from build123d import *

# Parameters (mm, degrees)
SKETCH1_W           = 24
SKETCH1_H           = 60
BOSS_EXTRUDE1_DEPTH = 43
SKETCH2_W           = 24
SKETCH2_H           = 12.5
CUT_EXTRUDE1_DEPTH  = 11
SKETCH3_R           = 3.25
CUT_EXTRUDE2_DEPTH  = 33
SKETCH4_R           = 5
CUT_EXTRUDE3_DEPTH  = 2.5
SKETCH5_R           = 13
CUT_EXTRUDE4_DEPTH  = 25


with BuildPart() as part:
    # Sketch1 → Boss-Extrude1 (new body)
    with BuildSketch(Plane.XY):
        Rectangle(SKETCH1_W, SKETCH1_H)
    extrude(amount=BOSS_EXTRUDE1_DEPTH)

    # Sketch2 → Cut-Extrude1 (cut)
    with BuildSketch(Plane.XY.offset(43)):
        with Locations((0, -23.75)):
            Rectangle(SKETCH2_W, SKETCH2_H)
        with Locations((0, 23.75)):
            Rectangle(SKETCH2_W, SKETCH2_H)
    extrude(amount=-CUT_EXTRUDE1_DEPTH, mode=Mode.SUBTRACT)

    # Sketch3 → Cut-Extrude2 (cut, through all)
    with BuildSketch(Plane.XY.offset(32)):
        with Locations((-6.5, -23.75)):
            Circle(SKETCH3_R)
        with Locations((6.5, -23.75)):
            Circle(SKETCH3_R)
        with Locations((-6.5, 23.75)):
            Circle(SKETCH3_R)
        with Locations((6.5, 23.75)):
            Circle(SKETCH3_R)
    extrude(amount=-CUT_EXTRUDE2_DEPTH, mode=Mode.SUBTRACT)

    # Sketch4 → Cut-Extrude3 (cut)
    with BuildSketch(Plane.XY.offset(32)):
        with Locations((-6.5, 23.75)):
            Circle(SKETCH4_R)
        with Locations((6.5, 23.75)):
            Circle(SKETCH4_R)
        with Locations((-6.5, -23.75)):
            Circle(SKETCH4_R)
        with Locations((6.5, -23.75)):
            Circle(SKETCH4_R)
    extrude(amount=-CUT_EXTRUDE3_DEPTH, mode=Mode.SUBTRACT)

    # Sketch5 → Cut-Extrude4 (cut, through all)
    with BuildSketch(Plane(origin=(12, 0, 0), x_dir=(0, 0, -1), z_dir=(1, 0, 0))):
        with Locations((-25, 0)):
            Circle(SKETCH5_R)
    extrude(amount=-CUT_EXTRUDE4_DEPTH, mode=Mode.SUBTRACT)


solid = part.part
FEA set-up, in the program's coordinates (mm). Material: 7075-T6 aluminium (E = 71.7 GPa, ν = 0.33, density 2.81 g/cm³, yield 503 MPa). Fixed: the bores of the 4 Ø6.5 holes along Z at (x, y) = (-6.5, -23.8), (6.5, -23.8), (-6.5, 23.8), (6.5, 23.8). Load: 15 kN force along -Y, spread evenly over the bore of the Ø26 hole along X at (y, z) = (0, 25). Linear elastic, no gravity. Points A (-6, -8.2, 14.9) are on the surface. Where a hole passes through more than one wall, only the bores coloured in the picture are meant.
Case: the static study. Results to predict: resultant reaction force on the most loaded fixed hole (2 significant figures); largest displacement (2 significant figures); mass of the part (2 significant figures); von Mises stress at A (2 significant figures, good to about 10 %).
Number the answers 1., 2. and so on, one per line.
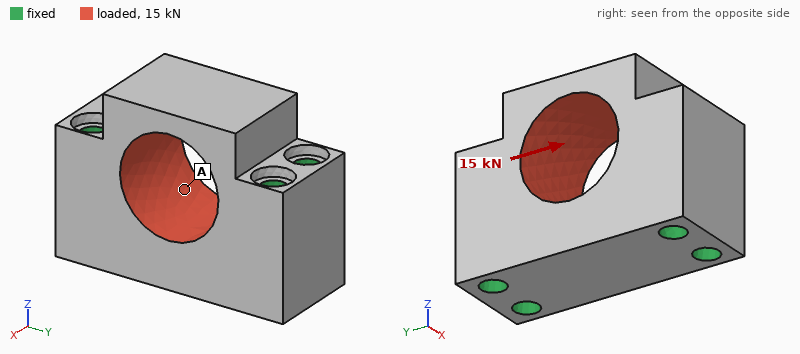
1. 3.9 kN
2. 16 µm
3. 110 g
4. 11 MPa
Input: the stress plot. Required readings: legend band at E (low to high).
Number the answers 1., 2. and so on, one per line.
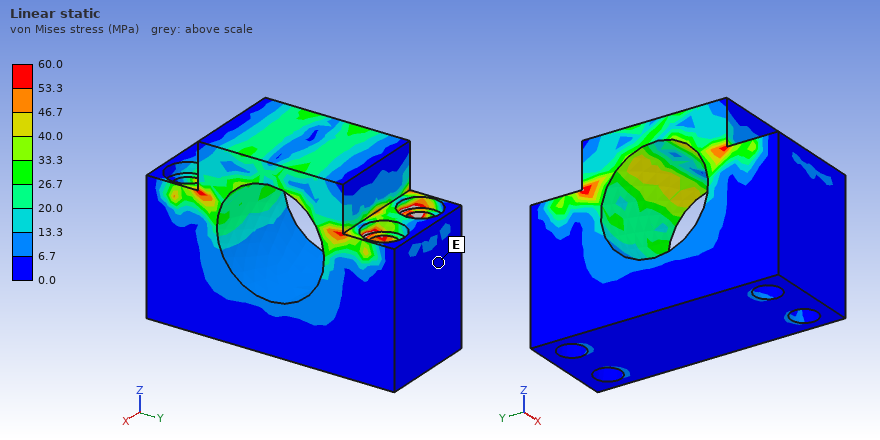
1. 0.0 to 6.7 MPa
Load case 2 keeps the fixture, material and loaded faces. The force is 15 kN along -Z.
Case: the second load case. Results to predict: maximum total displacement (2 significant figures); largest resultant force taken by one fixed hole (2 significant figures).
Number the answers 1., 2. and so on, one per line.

1. 14 µm
2. 3.8 kN
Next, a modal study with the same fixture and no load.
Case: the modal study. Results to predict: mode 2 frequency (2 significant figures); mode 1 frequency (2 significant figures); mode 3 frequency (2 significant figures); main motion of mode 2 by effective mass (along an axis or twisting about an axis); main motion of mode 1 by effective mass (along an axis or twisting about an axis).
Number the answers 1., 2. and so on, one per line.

1. 22 kHz
2. 19 kHz
3. 25 kHz
4. along Y
5. along X
